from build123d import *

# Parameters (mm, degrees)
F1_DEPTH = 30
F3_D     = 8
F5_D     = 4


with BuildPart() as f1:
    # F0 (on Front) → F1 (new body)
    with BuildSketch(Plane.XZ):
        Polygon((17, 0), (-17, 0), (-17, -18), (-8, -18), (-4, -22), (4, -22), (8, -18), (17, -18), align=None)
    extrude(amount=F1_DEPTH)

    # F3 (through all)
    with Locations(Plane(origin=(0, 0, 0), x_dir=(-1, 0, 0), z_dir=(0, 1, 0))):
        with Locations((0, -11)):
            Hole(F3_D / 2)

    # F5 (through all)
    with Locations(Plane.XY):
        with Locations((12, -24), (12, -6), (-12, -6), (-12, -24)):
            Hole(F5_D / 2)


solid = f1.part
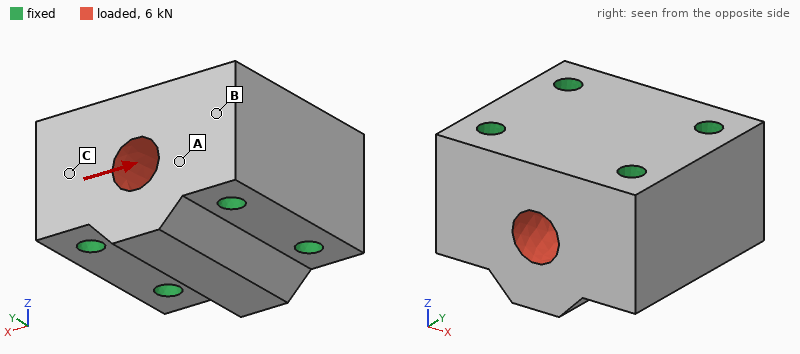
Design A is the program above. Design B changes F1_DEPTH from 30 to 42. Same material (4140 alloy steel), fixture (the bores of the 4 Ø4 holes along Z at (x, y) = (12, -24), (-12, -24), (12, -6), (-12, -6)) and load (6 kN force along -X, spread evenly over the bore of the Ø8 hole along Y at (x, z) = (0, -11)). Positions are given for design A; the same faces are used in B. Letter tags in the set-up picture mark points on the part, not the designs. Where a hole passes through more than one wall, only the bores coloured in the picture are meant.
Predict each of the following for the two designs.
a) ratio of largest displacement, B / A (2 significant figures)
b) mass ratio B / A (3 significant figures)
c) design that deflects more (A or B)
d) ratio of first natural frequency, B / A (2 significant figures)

2.0
1.42
B
0.49
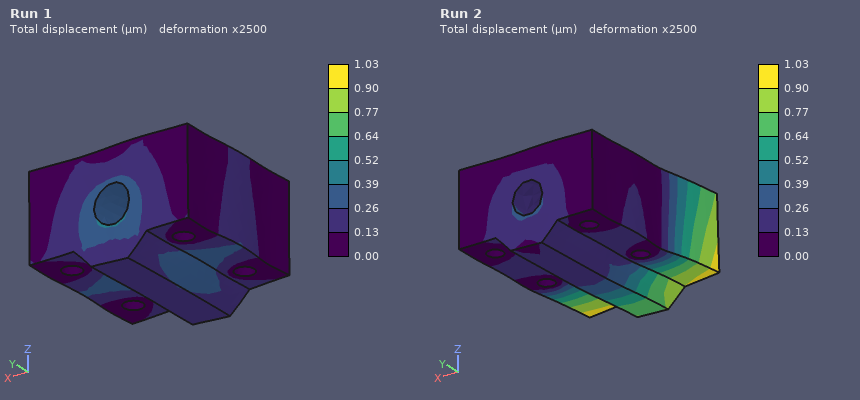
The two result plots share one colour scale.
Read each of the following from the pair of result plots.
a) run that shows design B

Run 2
